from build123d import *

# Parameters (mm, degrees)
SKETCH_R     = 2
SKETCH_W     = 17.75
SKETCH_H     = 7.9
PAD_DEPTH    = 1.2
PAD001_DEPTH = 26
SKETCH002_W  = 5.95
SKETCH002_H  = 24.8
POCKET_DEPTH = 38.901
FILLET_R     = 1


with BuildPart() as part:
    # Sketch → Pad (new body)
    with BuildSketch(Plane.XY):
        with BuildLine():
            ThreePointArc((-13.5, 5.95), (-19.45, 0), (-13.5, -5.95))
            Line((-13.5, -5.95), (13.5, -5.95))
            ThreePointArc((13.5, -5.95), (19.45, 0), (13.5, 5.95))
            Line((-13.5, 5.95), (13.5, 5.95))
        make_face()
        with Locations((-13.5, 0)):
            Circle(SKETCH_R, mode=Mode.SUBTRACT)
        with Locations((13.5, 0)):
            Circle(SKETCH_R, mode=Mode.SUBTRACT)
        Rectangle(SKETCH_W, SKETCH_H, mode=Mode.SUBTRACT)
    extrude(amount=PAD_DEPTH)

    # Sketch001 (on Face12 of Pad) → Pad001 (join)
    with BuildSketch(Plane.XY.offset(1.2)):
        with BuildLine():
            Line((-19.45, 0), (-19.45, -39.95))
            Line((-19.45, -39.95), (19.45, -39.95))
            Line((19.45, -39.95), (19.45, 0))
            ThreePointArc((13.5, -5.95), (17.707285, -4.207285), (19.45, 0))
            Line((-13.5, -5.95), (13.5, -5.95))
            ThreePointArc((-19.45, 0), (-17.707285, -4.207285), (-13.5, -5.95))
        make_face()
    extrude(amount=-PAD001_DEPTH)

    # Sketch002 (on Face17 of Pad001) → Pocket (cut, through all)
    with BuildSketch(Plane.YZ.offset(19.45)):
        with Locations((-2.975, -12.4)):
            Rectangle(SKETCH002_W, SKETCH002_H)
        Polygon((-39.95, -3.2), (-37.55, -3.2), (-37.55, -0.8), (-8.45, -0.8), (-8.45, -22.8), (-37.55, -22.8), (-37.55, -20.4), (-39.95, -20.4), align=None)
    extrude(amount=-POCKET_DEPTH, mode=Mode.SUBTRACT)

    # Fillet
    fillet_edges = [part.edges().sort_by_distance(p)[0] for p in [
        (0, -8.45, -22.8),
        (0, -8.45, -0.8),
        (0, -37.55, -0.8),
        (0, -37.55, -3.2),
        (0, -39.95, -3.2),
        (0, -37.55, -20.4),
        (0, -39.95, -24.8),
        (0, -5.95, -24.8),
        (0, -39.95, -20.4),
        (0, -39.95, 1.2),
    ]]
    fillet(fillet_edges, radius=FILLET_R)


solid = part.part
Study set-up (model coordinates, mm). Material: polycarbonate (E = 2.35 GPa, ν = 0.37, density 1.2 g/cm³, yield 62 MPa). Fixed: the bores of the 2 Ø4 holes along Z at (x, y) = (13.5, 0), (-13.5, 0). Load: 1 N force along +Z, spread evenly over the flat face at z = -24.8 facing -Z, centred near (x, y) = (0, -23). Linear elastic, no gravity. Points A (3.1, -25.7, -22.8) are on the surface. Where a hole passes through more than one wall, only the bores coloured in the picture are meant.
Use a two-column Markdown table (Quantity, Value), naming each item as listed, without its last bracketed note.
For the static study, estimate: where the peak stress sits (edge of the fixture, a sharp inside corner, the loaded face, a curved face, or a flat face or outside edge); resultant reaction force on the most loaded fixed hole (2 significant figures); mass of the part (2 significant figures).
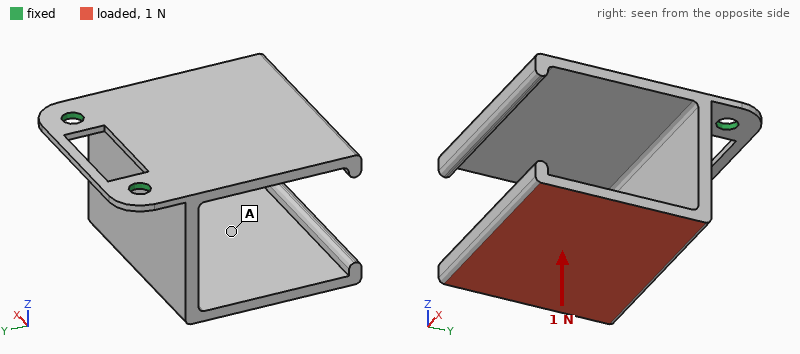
| Quantity | Value |
|---|---|
| where the peak stress sits | a flat face or outside edge |
| resultant reaction force on the most loaded fixed hole | 0.50 N |
| mass of the part | 9.8 g |
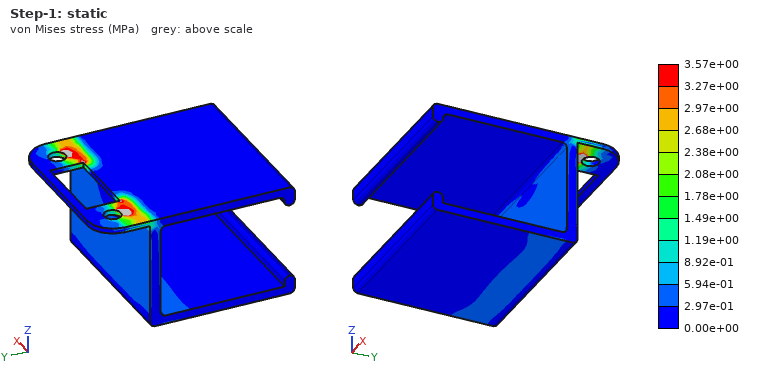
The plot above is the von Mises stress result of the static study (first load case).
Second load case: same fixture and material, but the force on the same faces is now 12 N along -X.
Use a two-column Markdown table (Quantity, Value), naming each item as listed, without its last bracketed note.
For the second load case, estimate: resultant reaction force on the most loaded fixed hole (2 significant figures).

| Quantity | Value |
|---|---|
| resultant reaction force on the most loaded fixed hole | 15 N |
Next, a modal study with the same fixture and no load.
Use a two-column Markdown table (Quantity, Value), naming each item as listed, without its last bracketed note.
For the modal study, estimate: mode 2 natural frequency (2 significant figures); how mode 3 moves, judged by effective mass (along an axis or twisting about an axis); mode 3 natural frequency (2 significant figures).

| Quantity | Value |
|---|---|
| mode 2 natural frequency | 310 Hz |
| how mode 3 moves, judged by effective mass | along X |
| mode 3 natural frequency | 370 Hz |
